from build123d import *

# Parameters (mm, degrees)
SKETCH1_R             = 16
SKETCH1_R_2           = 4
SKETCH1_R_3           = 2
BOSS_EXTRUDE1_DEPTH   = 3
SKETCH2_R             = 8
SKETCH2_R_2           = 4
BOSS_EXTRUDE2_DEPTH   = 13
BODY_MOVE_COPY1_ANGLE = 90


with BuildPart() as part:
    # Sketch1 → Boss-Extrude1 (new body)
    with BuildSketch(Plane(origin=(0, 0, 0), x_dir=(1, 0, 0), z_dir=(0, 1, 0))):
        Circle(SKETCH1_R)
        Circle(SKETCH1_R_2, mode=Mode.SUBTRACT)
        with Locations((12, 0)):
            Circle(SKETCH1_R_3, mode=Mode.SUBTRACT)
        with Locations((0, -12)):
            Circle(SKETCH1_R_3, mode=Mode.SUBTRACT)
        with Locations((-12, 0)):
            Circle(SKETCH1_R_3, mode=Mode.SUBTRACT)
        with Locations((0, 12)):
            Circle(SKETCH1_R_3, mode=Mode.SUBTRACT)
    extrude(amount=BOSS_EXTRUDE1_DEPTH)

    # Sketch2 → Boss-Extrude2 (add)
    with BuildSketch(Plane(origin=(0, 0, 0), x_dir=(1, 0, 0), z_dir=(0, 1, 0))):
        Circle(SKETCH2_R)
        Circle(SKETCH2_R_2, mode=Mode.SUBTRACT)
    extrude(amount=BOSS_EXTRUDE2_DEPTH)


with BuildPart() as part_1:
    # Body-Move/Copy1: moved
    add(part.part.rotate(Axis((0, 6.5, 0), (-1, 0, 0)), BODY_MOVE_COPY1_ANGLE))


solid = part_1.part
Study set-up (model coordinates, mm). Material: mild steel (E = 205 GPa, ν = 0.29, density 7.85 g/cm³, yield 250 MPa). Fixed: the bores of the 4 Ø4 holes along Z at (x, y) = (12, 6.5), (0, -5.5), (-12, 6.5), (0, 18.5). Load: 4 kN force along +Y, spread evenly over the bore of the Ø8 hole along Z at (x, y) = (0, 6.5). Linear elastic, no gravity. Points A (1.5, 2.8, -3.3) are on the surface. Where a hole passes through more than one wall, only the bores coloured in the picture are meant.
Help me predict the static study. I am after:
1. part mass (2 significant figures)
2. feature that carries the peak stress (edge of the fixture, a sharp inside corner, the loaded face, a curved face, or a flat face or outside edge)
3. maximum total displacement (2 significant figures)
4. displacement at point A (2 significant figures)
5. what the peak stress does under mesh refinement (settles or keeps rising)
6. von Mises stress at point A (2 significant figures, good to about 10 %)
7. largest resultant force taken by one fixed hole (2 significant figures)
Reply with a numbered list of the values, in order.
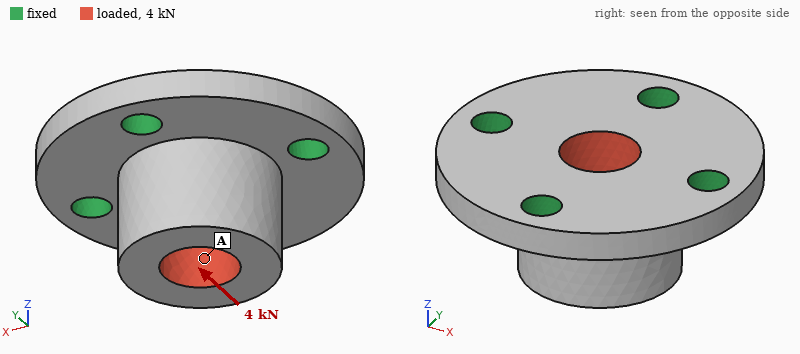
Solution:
1. 28 g
2. edge of the fixture
3. 8.3 µm
4. 6.0 µm
5. keeps rising
6. 23 MPa
7. 1.6 kN
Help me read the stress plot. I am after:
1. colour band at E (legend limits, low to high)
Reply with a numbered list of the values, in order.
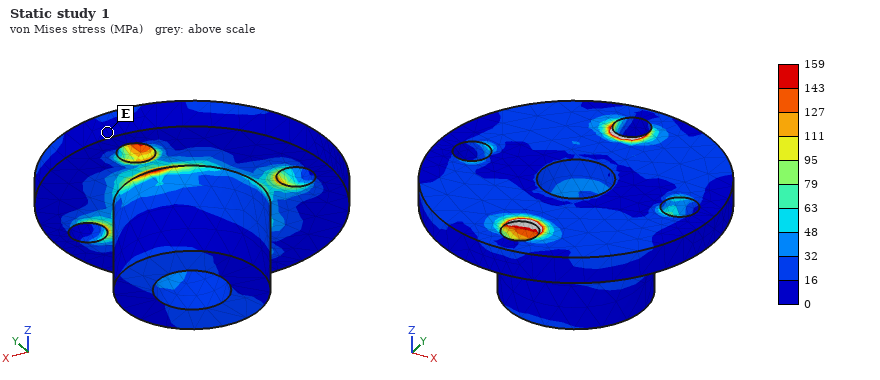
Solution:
1. 0 to 16 MPa
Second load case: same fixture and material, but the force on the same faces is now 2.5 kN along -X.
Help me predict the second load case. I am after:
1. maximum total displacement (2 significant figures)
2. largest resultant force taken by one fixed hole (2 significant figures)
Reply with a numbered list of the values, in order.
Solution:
1. 5.2 µm
2. 1.0 kN
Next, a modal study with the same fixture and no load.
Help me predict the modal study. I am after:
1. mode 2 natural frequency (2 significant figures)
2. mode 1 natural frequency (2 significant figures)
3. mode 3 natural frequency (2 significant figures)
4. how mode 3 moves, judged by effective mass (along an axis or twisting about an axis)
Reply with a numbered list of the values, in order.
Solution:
1. 31 kHz
2. 31 kHz
3. 38 kHz
4. along Z
